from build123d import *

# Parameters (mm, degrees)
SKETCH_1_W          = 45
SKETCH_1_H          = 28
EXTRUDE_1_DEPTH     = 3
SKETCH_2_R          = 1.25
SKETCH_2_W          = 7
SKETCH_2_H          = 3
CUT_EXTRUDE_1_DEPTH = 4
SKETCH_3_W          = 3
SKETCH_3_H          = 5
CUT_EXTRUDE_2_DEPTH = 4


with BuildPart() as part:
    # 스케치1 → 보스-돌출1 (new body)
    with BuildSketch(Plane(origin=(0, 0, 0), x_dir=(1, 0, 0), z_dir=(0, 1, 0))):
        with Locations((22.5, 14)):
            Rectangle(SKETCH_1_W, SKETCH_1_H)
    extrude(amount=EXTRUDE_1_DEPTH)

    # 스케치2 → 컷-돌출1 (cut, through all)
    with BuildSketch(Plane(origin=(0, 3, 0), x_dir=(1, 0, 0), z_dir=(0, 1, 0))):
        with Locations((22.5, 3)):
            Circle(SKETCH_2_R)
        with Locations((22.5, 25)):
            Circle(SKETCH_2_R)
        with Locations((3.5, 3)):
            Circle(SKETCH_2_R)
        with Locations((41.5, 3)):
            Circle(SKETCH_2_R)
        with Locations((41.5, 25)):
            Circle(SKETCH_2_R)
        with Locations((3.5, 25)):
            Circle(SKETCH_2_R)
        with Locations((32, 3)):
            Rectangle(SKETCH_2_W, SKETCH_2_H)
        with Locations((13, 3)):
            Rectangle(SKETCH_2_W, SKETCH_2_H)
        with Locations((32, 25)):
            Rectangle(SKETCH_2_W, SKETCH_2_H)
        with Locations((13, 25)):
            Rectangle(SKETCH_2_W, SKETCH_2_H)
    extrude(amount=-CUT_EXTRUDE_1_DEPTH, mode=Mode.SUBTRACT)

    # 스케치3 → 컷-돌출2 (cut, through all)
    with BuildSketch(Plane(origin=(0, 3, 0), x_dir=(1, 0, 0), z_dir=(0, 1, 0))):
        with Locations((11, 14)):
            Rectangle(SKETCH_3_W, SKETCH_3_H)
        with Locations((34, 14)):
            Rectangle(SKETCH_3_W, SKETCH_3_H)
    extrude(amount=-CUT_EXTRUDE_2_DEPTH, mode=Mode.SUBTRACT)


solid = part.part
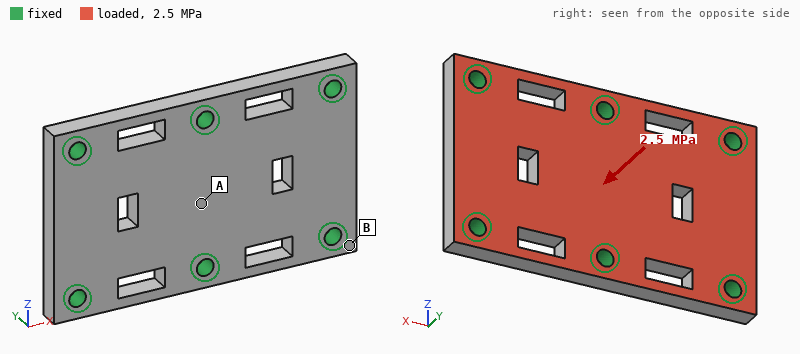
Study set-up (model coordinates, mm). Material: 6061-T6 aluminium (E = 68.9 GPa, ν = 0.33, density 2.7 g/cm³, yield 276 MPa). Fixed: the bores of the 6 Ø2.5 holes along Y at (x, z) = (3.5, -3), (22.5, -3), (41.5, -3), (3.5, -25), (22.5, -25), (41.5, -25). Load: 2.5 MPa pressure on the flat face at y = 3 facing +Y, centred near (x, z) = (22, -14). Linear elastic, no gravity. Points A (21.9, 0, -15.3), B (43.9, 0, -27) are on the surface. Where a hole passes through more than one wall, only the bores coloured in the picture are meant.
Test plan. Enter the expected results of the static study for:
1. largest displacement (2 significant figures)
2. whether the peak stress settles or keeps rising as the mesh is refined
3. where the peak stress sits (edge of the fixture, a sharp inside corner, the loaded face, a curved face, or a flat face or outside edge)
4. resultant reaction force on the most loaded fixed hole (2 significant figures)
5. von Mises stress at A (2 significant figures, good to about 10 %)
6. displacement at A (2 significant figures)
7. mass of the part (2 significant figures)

21 µm
keeps rising
edge of the fixture
600 N
40 MPa
16 µm
9.0 g
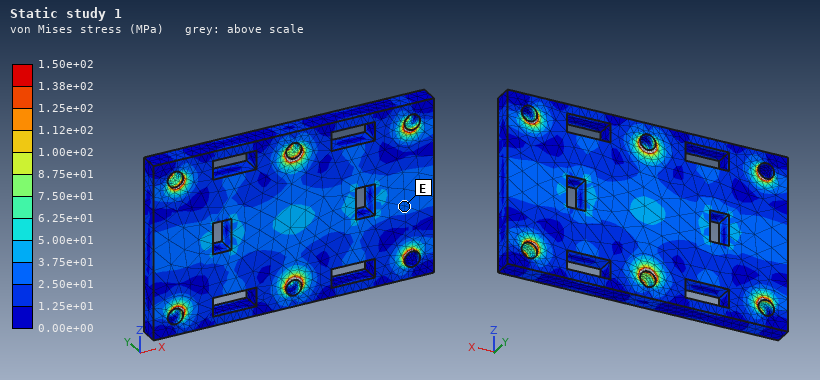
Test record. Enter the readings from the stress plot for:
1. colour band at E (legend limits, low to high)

2.50e+01 to 3.75e+01 MPa
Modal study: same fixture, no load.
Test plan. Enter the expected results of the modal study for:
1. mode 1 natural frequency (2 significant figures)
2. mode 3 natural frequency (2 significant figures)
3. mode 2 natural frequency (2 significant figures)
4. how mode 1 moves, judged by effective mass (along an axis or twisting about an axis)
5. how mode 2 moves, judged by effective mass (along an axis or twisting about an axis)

24 kHz
35 kHz
26 kHz
along Y
twisting about Z
